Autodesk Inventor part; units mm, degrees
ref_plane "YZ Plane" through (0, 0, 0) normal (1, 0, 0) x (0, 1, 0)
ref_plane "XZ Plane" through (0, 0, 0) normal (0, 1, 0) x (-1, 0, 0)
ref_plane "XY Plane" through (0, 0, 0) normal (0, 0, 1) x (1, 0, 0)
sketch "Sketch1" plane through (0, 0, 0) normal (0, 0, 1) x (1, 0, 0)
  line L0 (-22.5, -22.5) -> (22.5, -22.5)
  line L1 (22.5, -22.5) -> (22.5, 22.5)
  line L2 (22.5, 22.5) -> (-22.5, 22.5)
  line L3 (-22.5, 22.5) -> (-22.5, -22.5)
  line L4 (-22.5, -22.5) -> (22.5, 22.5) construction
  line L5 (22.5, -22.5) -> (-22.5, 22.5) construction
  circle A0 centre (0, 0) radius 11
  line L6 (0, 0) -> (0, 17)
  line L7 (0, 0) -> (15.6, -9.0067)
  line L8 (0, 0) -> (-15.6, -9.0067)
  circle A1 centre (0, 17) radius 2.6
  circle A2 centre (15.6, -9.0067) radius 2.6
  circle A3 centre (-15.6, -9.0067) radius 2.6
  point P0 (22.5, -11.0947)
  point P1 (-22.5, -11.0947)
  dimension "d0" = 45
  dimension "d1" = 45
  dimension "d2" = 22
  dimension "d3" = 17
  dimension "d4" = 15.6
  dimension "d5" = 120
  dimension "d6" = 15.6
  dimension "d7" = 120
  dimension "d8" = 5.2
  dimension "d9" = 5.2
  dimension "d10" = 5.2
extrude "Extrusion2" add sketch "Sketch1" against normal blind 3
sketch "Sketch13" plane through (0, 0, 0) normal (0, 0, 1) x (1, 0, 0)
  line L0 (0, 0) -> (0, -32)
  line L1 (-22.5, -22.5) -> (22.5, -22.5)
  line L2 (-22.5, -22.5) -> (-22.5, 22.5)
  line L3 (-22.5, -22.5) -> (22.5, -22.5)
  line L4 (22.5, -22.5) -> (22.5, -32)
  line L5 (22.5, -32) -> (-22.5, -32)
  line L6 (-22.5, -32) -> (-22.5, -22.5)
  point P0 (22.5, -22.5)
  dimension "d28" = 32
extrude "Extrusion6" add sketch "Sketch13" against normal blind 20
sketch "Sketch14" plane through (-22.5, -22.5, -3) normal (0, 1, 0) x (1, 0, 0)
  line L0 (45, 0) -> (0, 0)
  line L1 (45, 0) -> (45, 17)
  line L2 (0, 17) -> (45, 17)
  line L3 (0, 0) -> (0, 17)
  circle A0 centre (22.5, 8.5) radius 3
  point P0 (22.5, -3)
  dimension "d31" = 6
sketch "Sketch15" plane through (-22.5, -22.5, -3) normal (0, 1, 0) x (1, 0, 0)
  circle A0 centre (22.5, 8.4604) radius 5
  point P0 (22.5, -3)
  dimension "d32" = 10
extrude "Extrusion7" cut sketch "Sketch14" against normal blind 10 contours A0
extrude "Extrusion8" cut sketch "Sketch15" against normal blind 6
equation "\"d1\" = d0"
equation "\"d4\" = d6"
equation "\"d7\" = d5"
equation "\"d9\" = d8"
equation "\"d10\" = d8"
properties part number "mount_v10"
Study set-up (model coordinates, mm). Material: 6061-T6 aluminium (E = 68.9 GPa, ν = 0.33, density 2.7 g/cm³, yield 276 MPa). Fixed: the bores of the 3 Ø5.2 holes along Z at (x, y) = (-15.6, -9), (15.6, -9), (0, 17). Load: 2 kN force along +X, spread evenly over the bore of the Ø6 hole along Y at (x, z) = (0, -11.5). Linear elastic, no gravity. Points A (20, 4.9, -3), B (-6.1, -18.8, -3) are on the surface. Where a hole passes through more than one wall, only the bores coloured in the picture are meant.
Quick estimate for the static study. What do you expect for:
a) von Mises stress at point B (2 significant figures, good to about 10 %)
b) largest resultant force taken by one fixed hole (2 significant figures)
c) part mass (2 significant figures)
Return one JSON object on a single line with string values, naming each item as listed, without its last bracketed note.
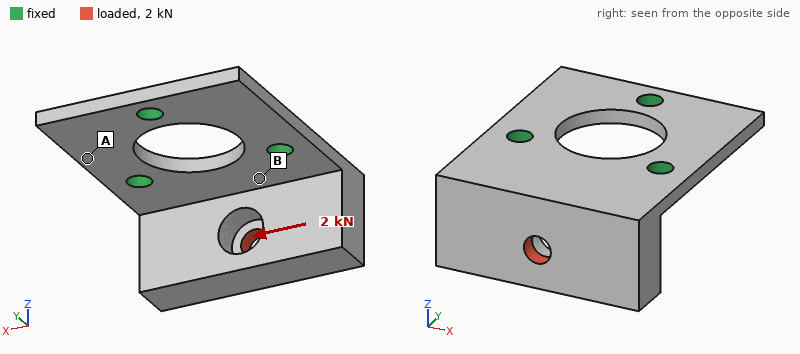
{"von Mises stress at point B": "79 MPa", "largest resultant force taken by one fixed hole": "1.7 kN", "part mass": "34 g"}
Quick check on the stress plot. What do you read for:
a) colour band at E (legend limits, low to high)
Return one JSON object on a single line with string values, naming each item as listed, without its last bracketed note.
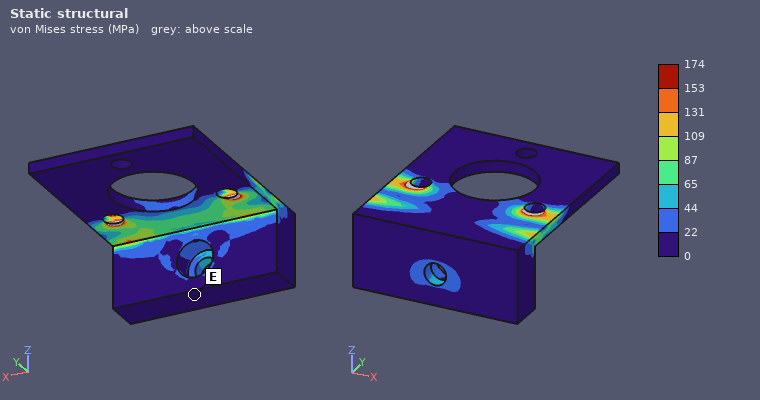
{"colour band at E": "0 to 22 MPa"}
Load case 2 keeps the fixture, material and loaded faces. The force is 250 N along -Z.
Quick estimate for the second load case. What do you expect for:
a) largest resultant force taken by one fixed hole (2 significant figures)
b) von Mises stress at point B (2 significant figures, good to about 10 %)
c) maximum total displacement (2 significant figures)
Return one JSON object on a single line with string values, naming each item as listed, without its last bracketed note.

{"largest resultant force taken by one fixed hole": "130 N", "von Mises stress at point B": "34 MPa", "maximum total displacement": "0.18 mm"}
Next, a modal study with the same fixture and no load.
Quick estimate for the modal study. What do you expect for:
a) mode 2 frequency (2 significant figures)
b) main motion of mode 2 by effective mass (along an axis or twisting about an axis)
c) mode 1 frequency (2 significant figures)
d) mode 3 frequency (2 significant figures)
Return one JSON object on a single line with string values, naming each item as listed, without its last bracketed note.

{"mode 2 frequency": "4300 Hz", "main motion of mode 2 by effective mass": "along X", "mode 1 frequency": "1500 Hz", "mode 3 frequency": "7000 Hz"}
